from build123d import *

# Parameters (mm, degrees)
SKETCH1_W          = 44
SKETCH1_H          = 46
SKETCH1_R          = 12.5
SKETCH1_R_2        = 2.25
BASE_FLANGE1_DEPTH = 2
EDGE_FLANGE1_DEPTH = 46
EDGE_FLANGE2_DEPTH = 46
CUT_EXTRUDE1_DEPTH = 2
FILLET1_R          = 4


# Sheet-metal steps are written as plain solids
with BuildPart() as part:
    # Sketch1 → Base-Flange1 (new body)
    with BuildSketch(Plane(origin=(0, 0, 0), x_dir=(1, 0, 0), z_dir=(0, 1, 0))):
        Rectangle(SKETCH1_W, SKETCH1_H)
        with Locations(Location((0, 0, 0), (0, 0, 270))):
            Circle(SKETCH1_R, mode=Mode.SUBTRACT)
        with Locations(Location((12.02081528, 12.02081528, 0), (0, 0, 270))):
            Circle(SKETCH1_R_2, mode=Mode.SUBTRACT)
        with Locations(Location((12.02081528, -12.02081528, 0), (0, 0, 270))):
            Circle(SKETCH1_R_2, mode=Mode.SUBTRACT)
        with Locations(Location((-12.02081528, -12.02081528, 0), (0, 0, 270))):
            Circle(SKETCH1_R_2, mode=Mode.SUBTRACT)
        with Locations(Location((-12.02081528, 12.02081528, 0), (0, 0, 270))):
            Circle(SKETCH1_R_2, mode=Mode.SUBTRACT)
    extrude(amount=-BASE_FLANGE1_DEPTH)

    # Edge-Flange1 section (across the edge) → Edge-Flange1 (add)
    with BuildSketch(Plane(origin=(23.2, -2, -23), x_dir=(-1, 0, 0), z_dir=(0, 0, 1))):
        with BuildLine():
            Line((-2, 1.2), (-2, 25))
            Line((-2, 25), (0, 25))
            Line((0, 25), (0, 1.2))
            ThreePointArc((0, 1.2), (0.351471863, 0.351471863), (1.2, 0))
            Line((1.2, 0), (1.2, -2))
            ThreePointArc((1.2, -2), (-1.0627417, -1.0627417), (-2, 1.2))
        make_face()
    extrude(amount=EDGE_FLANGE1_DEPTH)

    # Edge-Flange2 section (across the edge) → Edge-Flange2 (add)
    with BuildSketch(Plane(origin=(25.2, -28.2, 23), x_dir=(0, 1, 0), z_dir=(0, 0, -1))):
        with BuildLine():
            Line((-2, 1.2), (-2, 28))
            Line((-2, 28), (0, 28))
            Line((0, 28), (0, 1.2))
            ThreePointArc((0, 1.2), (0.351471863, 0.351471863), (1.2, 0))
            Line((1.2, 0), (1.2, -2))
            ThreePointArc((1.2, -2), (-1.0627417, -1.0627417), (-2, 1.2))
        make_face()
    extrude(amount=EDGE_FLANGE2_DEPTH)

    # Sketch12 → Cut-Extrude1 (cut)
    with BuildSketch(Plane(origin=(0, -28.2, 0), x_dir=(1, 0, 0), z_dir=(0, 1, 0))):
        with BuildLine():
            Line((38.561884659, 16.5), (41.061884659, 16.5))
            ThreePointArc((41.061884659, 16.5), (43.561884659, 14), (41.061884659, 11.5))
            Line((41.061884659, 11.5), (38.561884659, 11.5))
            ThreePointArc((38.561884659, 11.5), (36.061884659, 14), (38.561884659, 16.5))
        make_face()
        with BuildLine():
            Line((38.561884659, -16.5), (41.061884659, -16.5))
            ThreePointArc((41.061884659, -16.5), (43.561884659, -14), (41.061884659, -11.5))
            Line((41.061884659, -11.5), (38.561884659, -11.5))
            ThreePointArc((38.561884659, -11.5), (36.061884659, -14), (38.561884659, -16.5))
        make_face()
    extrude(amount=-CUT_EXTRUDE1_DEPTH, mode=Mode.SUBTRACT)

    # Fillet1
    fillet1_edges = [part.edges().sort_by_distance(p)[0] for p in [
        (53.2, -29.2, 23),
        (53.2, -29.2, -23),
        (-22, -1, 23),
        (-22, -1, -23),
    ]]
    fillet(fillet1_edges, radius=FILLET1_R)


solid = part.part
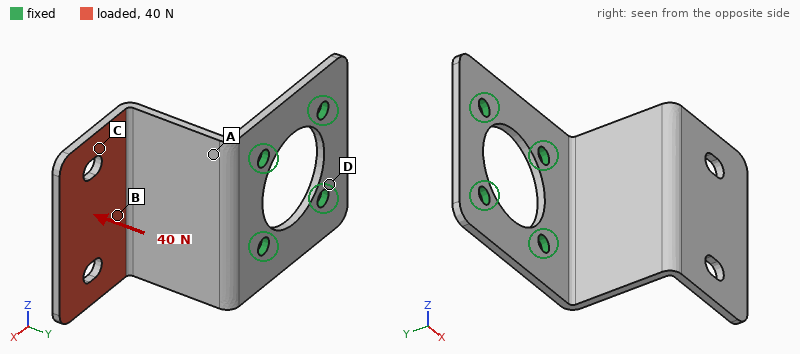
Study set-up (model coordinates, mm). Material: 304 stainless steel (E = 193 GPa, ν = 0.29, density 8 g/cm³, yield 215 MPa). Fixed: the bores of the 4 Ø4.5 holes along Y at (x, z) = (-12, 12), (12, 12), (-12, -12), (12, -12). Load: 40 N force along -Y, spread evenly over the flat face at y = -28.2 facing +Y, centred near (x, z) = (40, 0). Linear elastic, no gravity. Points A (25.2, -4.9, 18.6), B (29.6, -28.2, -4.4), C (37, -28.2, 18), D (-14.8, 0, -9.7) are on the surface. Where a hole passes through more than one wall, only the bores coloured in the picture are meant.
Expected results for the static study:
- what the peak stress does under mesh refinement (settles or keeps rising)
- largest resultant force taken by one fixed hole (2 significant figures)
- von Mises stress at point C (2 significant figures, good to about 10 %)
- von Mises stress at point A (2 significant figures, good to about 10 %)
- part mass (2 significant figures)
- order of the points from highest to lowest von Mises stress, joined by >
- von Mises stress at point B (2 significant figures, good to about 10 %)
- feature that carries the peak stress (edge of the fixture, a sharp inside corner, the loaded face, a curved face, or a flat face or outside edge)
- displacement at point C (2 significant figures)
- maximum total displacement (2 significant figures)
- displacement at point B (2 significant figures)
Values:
keeps rising
22 N
8.4 MPa
18 MPa
65 g
A > B > C > D
13 MPa
edge of the fixture
0.11 mm
0.18 mm
0.087 mm
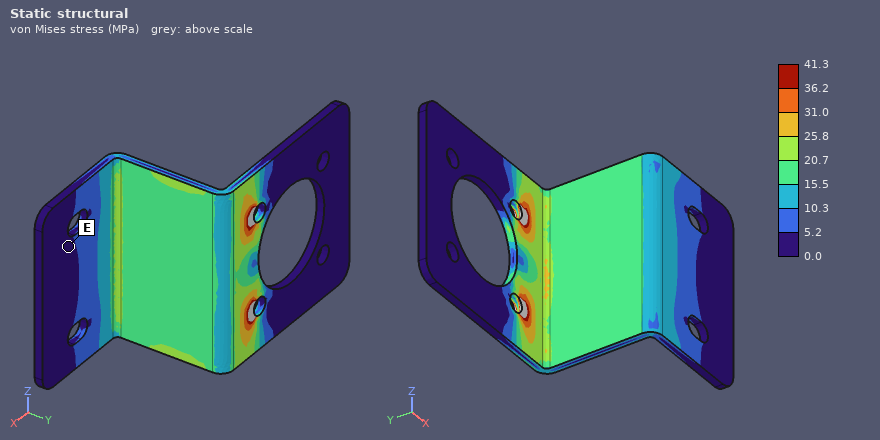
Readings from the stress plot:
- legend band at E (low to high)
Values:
0.0 to 5.2 MPa
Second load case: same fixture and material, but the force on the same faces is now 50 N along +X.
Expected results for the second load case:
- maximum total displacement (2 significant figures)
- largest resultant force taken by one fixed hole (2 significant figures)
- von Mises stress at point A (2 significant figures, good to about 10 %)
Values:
0.21 mm
27 N
33 MPa
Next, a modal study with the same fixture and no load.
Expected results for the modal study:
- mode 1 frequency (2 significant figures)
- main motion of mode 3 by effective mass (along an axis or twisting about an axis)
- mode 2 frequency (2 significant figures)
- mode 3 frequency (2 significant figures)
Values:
480 Hz
along X
1200 Hz
1700 Hz
